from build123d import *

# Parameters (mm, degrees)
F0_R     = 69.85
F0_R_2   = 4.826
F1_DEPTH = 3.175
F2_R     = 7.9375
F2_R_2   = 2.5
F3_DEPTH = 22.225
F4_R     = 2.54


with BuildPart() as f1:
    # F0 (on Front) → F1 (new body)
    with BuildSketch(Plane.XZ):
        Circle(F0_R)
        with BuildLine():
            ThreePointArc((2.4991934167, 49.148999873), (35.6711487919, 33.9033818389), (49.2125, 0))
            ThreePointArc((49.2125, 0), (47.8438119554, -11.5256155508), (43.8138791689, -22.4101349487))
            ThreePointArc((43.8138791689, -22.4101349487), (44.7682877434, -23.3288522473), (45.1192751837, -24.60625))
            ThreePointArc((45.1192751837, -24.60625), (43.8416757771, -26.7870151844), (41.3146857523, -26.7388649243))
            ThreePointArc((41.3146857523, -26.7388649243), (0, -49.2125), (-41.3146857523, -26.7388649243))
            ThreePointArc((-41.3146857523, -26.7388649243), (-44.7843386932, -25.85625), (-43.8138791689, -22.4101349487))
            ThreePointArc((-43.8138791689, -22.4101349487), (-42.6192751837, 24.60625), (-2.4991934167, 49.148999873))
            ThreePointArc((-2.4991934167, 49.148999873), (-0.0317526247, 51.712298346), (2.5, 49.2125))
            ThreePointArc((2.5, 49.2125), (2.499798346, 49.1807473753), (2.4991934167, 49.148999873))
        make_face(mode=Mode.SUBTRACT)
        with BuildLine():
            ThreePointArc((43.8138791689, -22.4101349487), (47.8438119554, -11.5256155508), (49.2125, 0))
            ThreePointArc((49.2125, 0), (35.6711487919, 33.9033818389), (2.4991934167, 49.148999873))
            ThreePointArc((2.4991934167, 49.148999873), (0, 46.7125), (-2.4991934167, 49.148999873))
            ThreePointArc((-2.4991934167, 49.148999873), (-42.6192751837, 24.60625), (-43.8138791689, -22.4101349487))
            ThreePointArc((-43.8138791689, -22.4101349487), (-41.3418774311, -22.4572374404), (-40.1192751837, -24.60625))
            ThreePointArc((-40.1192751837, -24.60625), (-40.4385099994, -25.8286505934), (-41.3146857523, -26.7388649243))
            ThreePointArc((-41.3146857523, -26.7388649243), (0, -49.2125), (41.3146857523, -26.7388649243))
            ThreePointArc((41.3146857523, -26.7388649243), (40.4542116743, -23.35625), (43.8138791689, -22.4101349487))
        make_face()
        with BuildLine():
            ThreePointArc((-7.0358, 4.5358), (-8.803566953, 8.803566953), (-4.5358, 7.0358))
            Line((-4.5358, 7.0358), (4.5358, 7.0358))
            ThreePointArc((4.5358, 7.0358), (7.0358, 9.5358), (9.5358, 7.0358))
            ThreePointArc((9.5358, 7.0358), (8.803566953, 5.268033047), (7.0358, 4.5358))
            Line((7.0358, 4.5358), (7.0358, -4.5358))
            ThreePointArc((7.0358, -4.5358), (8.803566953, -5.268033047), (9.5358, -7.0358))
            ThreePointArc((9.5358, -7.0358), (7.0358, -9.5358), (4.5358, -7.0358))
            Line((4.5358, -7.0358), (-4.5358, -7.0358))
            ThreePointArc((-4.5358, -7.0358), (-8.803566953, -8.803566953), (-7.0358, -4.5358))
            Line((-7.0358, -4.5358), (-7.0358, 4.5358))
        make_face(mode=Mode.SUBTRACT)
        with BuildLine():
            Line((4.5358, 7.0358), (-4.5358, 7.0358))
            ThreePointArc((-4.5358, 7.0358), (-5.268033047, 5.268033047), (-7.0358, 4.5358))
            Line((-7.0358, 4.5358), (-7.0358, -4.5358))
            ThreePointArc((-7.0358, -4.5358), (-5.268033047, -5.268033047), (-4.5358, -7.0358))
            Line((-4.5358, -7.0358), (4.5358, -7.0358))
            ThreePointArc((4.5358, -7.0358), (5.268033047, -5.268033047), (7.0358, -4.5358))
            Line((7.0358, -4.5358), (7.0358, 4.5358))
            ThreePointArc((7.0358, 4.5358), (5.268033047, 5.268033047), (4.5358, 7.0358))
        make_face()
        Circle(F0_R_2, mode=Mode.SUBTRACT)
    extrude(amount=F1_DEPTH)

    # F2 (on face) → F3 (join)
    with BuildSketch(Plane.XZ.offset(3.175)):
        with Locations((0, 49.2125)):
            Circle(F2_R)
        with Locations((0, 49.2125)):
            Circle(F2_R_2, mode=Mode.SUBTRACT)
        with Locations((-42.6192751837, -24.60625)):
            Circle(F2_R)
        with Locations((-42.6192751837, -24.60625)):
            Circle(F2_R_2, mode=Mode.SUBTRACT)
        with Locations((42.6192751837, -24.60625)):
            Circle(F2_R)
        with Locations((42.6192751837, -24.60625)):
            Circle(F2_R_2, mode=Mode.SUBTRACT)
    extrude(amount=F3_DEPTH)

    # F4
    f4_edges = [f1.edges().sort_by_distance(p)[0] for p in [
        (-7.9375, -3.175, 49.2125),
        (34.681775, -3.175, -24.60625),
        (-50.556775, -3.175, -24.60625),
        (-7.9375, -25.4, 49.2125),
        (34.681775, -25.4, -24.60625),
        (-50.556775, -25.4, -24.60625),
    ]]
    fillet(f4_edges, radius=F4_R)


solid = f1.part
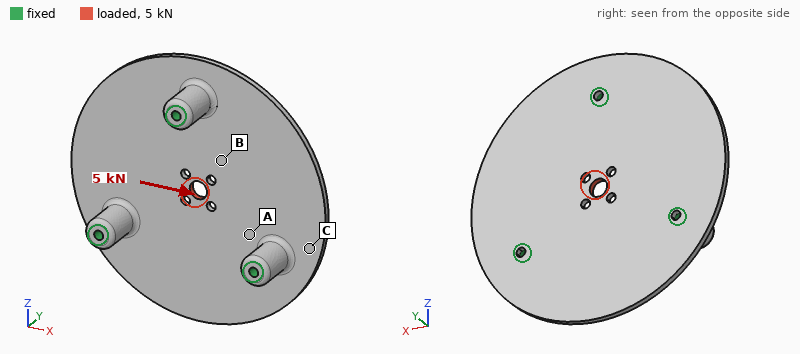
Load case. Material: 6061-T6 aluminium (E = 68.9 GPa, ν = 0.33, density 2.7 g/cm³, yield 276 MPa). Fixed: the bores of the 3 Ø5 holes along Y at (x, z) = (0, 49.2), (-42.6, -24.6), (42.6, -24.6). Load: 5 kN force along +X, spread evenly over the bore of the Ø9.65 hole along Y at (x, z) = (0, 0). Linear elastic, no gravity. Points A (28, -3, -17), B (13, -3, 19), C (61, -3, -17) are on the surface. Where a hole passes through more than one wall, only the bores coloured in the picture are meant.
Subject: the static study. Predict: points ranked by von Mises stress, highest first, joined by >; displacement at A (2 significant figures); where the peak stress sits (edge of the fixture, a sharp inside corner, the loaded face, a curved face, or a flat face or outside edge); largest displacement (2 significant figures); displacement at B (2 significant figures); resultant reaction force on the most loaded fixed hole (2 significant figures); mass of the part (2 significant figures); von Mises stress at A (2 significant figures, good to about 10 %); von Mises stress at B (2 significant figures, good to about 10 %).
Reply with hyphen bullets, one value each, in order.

- A > B > C
- 7.7 µm
- a curved face
- 25 µm
- 11 µm
- 1.8 kN
- 160 g
- 24 MPa
- 12 MPa
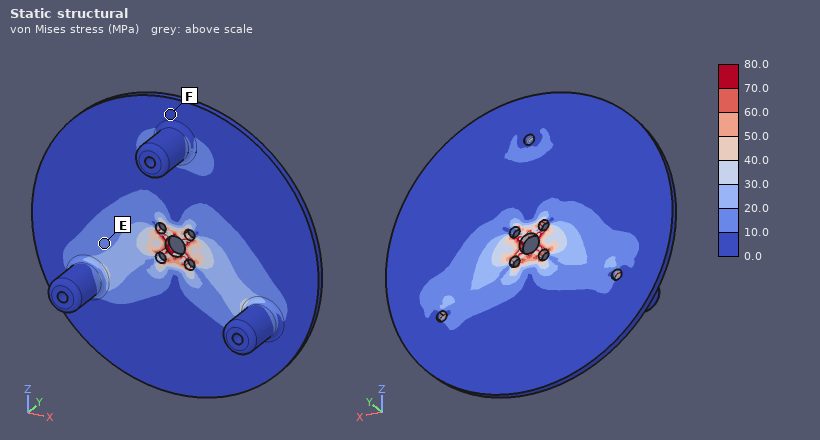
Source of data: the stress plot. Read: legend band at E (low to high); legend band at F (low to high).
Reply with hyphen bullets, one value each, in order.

- 10.0 to 20.0 MPa
- 0.0 to 10.0 MPa
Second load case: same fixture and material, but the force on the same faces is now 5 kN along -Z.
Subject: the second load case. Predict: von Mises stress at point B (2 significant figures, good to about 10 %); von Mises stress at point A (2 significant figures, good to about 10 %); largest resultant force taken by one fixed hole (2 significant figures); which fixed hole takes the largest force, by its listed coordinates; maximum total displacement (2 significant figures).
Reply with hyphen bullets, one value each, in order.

- 17 MPa
- 15 MPa
- 1.9 kN
- (0, 49.2)
- 25 µm
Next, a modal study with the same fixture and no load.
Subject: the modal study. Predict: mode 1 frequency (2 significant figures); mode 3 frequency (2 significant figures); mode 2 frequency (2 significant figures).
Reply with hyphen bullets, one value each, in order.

- 1500 Hz
- 1500 Hz
- 1500 Hz
